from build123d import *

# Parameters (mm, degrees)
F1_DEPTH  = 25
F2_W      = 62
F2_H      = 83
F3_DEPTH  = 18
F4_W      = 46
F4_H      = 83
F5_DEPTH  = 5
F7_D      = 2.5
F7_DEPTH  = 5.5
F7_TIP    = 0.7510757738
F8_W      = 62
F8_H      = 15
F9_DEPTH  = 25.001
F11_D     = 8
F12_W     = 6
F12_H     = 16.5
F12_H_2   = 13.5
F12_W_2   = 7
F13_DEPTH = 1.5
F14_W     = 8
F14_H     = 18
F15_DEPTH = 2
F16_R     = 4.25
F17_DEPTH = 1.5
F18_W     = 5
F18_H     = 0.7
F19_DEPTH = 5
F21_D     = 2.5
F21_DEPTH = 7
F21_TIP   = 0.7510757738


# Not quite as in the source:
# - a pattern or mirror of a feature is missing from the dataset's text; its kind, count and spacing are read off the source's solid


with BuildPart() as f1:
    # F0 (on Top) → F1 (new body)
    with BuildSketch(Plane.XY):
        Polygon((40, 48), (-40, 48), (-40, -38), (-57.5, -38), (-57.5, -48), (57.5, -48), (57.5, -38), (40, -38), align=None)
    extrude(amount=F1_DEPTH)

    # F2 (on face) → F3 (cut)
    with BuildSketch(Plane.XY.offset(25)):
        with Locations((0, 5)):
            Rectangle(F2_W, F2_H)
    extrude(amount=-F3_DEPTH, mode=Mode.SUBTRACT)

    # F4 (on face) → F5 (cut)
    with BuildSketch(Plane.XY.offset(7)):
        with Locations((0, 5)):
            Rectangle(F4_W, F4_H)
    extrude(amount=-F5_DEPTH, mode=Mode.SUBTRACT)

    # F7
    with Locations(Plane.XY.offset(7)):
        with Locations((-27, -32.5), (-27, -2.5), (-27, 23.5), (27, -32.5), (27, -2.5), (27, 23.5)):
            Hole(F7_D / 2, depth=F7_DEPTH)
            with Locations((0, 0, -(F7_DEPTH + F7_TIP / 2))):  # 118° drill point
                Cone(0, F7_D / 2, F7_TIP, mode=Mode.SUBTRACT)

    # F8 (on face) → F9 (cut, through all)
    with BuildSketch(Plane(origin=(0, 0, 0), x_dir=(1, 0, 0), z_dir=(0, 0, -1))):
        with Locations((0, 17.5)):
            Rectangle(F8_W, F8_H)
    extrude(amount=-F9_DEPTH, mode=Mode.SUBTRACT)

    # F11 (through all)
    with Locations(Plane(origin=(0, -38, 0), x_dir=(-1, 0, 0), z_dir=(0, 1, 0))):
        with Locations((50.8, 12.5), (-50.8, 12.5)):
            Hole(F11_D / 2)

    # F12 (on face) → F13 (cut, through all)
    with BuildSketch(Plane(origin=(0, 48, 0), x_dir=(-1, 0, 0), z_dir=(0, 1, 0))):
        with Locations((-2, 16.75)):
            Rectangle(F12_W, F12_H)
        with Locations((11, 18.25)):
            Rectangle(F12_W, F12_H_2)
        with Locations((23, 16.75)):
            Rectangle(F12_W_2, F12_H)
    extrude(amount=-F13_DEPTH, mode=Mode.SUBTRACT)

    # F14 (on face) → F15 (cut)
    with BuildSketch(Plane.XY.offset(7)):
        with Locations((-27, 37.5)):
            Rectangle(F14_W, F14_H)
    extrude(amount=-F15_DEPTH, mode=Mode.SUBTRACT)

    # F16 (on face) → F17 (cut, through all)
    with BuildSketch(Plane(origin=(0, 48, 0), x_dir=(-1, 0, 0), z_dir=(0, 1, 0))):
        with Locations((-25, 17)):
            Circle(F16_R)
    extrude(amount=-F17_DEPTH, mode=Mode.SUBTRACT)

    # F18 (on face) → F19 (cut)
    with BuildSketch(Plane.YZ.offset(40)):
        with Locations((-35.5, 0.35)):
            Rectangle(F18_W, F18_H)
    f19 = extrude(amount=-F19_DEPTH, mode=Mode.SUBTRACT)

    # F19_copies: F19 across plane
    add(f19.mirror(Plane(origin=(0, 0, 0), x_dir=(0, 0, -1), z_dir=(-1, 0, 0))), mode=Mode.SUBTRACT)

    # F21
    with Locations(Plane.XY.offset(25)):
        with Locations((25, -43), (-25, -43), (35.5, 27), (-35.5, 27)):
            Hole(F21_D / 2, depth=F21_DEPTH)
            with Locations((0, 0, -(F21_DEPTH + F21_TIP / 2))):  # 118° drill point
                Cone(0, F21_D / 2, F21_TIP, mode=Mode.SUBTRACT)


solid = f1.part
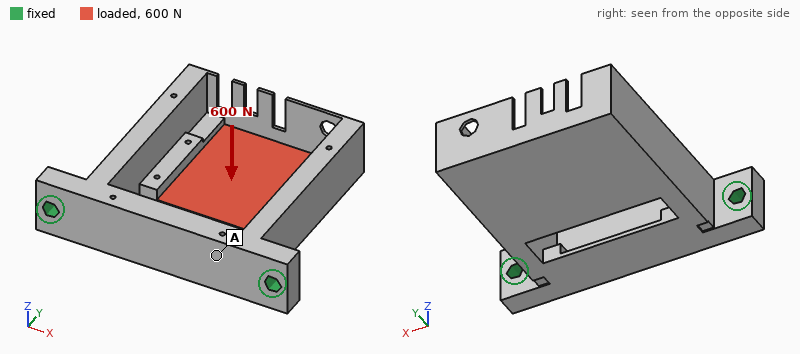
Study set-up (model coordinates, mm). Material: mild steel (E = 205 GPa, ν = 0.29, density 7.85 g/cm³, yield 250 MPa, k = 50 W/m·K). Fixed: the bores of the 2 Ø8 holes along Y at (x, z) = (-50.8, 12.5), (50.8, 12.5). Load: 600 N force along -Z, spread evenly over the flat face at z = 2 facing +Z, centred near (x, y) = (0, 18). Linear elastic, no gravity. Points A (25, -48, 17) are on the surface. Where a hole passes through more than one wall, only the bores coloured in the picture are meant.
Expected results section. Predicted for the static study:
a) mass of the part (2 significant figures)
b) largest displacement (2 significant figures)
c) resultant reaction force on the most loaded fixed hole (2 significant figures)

660 g
65 µm
300 N
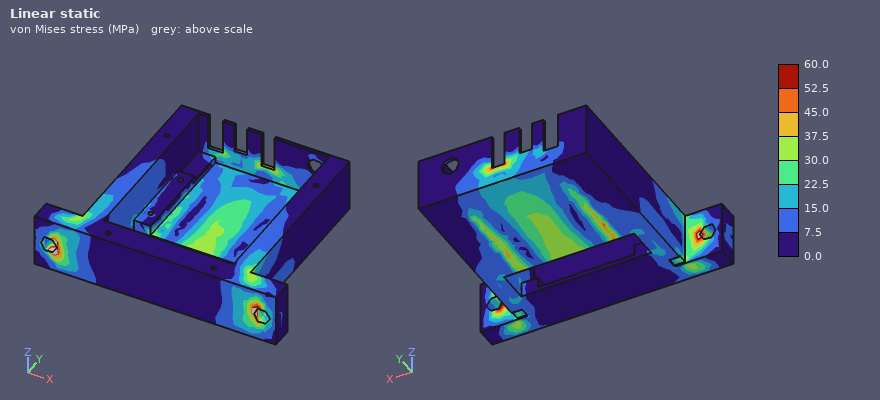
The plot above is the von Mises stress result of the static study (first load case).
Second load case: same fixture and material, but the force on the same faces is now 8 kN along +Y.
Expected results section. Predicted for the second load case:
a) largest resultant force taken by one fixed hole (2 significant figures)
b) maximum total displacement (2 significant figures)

4.1 kN
0.14 mm
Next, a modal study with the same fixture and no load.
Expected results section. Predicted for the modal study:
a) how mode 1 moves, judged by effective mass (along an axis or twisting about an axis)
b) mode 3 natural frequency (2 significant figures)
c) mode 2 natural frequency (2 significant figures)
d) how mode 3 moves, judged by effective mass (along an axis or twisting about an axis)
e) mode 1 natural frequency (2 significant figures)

along Z
2900 Hz
1600 Hz
along X
1100 Hz
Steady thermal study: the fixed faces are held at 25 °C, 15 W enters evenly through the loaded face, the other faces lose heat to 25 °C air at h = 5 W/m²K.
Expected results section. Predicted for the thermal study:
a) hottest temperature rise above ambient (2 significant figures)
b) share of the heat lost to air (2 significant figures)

49 K
21 %
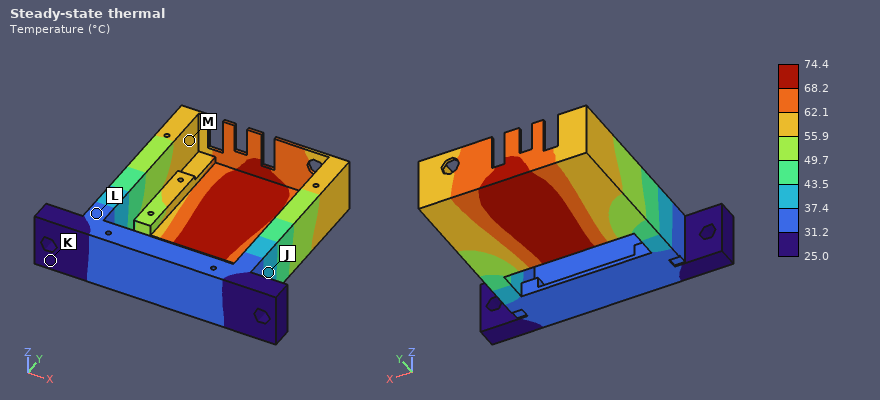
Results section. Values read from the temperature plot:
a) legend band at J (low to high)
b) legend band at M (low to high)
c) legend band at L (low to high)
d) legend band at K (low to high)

37.4 to 43.5 °C
55.9 to 62.1 °C
31.2 to 37.4 °C
25.0 to 31.2 °C
